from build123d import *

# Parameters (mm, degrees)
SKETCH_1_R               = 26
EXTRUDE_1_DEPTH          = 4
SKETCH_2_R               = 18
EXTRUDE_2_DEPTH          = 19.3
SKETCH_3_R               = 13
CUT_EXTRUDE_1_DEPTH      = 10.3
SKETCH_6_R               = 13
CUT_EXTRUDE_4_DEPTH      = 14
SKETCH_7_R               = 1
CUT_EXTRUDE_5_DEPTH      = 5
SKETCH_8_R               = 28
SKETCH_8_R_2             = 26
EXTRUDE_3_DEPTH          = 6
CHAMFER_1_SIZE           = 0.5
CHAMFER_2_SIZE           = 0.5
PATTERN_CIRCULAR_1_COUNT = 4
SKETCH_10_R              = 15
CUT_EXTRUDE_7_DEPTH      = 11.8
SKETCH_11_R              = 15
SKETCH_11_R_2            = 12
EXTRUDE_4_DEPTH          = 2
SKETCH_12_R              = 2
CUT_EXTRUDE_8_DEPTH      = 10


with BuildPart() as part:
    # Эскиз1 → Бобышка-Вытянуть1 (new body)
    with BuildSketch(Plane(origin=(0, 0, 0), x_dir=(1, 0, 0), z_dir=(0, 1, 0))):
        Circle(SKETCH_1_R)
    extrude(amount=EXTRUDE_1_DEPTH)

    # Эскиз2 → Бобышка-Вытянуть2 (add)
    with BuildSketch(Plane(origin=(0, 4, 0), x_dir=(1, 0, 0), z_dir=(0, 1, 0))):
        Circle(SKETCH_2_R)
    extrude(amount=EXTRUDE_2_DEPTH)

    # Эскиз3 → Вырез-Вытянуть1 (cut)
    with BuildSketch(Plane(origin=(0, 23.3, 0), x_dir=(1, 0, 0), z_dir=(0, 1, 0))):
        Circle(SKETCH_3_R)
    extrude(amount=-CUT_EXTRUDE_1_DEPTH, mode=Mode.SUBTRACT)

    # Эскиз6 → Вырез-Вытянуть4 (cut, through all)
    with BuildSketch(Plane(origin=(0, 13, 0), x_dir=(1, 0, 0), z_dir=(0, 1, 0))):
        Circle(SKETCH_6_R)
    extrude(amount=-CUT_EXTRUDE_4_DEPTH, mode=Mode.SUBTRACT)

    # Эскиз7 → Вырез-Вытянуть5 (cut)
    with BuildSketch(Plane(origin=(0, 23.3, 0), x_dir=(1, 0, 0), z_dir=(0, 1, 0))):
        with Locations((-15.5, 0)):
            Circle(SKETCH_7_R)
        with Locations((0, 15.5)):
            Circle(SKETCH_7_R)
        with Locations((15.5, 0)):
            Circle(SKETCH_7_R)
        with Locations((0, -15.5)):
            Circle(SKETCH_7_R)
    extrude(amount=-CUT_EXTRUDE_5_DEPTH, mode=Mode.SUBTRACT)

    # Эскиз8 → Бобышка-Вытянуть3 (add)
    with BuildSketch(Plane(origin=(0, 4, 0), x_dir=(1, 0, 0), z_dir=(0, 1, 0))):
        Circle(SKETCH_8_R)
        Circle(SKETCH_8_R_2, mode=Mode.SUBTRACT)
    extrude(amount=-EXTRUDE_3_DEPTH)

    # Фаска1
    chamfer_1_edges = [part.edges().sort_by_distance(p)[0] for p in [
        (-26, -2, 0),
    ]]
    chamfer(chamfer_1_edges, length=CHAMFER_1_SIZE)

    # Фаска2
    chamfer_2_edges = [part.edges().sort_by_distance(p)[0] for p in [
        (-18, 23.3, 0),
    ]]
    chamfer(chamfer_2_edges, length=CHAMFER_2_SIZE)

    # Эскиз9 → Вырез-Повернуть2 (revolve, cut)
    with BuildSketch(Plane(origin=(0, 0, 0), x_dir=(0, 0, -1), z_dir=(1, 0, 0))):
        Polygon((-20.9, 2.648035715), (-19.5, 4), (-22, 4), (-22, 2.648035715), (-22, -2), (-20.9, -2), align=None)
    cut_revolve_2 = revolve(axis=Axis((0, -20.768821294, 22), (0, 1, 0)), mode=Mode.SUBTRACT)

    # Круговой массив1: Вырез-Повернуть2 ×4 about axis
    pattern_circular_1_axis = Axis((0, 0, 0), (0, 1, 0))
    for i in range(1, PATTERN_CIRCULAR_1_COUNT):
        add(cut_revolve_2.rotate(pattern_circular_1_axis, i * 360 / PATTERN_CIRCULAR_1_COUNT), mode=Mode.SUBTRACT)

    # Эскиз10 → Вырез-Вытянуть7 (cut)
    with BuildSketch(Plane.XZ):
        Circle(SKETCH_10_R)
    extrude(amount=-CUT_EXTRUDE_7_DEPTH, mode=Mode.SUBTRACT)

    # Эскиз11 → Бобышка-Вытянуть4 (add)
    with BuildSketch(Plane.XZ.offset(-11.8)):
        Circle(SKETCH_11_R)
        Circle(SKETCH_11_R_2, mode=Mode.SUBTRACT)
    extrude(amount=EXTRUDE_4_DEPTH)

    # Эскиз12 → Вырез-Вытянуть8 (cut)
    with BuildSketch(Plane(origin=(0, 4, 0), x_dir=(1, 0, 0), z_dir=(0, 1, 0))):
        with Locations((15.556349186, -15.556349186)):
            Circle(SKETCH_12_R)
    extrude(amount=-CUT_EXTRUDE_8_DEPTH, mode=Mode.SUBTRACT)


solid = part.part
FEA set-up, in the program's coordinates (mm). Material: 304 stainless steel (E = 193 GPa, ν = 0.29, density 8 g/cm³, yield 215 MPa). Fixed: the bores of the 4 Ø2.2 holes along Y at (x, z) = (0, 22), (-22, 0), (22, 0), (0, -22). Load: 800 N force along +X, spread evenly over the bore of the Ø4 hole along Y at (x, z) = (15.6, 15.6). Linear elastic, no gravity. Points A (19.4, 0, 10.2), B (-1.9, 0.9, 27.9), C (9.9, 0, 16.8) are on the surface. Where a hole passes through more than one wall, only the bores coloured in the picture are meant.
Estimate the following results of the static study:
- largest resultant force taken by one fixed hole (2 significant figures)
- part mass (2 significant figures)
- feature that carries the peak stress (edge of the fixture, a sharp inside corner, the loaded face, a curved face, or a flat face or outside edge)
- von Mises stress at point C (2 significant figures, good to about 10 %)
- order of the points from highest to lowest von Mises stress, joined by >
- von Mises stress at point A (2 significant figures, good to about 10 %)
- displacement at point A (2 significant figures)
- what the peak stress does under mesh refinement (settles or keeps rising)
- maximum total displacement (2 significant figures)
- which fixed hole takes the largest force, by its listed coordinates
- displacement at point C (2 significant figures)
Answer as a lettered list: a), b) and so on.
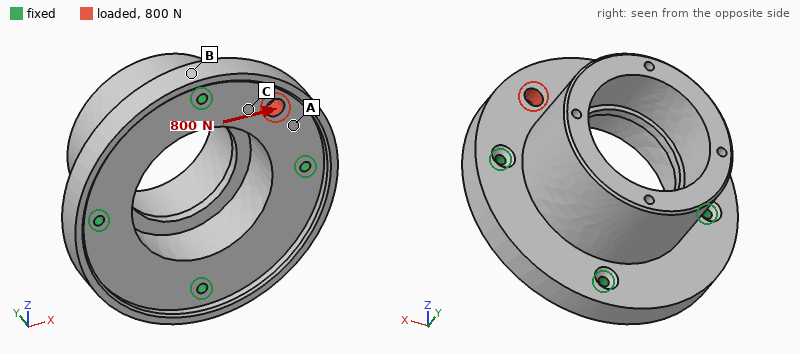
a) 580 N
b) 130 g
c) edge of the fixture
d) 19 MPa
e) C > A > B
f) 8.7 MPa
g) 1.4 µm
h) keeps rising
i) 2.1 µm
j) (0, 22)
k) 1.4 µm
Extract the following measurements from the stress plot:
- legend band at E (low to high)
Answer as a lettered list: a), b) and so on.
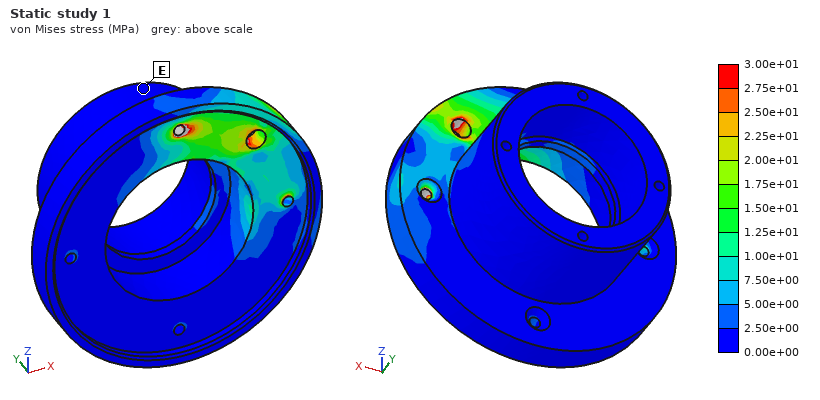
a) 0.00e+00 to 2.50e+00 MPa
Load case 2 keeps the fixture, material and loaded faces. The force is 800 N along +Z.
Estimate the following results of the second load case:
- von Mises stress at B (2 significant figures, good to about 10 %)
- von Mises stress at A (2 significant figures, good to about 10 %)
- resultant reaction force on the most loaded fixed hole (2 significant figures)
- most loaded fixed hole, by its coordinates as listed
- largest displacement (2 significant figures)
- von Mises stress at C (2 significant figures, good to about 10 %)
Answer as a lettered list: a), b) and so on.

a) 5.6 MPa
b) 17 MPa
c) 580 N
d) (22, 0)
e) 2.1 µm
f) 7.8 MPa
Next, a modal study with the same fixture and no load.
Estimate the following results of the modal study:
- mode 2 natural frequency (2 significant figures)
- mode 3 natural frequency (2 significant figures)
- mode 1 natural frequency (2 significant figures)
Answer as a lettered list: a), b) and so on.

a) 11 kHz
b) 12 kHz
c) 11 kHz
